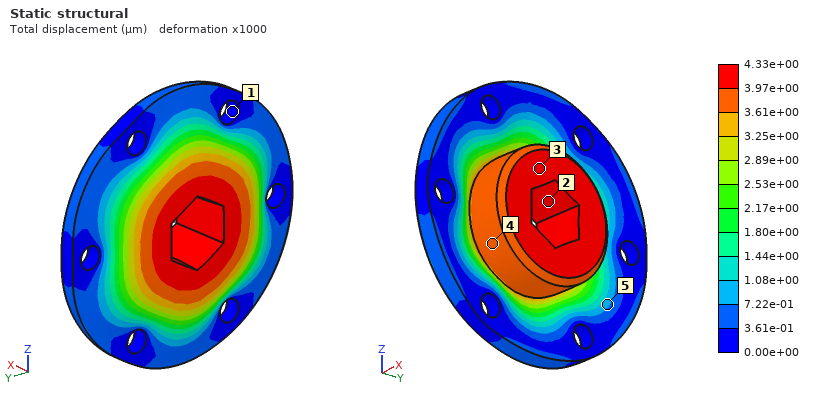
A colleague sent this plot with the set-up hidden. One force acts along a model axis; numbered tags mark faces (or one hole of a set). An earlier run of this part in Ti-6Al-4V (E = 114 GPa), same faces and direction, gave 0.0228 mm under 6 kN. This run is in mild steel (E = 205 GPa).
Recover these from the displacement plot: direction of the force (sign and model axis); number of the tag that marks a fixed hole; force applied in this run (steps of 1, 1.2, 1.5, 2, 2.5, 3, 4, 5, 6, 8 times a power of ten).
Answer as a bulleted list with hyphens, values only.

- -X
- 1
- 2 kN
